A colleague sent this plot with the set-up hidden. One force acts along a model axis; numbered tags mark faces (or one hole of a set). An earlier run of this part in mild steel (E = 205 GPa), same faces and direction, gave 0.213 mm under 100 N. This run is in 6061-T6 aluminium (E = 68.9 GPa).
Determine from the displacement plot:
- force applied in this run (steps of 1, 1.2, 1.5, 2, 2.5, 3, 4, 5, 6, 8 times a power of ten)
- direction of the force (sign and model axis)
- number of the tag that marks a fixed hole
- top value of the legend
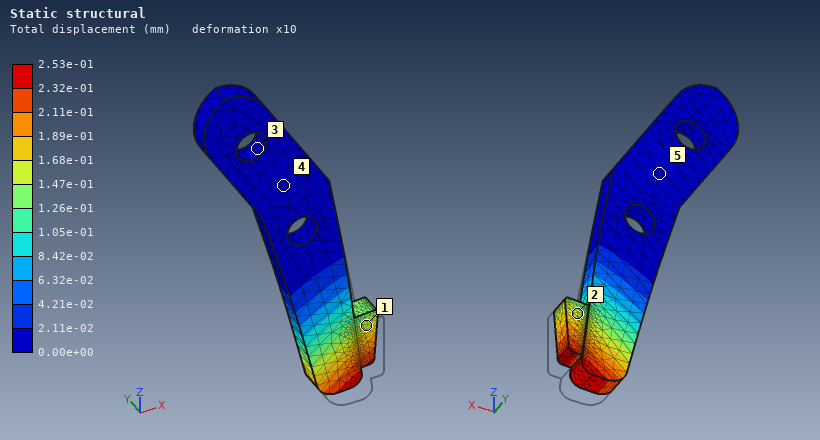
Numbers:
40 N
+Y
3
2.53e-01 mm
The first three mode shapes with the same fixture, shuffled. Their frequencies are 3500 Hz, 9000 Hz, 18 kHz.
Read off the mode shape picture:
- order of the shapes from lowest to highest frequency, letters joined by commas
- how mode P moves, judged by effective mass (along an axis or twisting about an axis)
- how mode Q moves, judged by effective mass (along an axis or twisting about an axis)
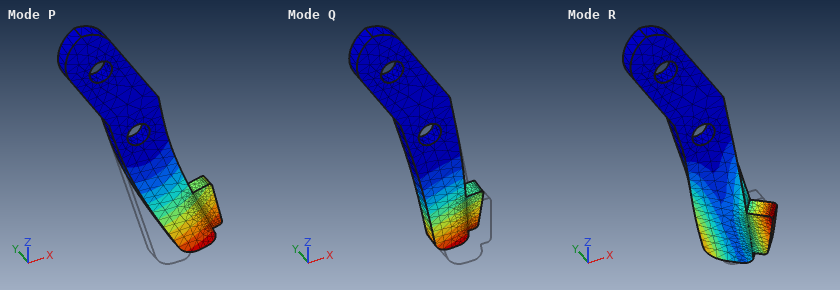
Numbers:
Q, P, R
along X
along Y
